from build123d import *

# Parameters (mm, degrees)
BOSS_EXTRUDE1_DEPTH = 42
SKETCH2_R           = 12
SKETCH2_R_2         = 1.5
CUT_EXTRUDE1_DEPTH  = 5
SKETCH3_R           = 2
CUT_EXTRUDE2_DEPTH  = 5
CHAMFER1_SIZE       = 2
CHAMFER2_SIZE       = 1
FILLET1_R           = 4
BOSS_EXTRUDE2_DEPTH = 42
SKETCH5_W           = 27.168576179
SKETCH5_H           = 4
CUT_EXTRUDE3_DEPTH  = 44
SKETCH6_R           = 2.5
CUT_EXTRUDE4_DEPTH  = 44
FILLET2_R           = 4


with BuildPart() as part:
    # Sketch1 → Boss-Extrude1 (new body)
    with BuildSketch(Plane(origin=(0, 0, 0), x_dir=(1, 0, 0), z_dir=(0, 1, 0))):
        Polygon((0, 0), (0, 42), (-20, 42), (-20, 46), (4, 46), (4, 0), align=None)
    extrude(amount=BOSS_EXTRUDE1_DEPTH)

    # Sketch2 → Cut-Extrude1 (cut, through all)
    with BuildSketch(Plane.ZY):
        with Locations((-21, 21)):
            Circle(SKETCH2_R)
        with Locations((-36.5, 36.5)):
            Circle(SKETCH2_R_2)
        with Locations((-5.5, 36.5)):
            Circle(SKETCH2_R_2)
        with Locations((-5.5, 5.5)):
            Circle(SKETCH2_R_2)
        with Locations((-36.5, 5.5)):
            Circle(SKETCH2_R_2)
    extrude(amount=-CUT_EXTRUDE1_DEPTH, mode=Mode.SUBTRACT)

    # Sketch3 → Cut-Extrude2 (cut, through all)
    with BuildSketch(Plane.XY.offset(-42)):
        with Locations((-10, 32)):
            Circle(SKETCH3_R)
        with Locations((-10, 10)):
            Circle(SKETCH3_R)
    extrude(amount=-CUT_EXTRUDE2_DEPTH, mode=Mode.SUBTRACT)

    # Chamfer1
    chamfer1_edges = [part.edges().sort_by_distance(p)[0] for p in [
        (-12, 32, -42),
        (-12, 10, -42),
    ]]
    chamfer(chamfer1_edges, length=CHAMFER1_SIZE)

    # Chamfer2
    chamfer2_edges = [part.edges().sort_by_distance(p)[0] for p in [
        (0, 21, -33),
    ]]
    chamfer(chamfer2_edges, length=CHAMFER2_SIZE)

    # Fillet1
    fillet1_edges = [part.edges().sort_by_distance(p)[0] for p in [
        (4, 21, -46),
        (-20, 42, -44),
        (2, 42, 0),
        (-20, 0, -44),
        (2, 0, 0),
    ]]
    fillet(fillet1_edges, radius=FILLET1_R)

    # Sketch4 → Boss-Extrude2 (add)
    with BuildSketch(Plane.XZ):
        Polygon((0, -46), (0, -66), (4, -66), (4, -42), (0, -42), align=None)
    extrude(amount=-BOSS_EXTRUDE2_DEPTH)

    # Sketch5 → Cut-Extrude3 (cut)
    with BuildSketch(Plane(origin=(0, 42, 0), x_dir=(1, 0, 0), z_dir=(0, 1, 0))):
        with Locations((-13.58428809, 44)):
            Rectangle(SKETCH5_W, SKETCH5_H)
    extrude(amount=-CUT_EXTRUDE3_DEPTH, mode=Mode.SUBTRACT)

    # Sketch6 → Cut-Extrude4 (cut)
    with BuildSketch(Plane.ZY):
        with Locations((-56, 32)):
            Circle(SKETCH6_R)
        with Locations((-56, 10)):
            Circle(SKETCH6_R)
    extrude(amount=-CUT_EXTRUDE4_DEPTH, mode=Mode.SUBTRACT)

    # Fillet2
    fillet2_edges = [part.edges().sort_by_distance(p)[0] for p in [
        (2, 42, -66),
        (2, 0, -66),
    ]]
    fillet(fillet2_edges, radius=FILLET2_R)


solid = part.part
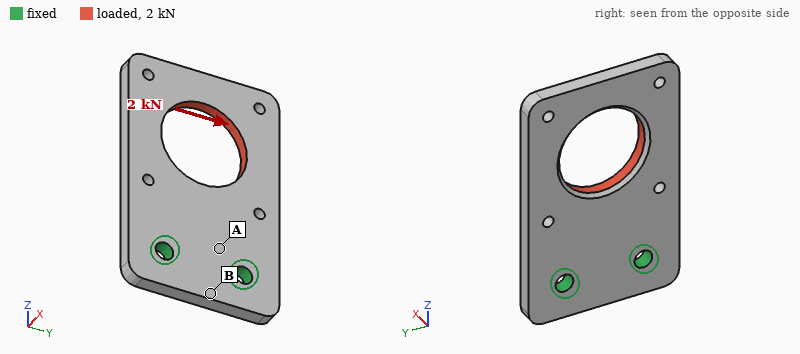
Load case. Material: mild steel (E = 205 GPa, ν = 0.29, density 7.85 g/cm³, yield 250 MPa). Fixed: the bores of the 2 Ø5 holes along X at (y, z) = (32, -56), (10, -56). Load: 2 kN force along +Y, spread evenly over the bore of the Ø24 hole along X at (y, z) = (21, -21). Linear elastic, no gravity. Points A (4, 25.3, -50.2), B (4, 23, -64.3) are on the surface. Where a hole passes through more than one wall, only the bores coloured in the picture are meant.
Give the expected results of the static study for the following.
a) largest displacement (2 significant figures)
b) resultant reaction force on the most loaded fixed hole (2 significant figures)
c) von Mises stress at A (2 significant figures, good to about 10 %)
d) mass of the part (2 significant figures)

40 µm
2.9 kN
44 MPa
70 g
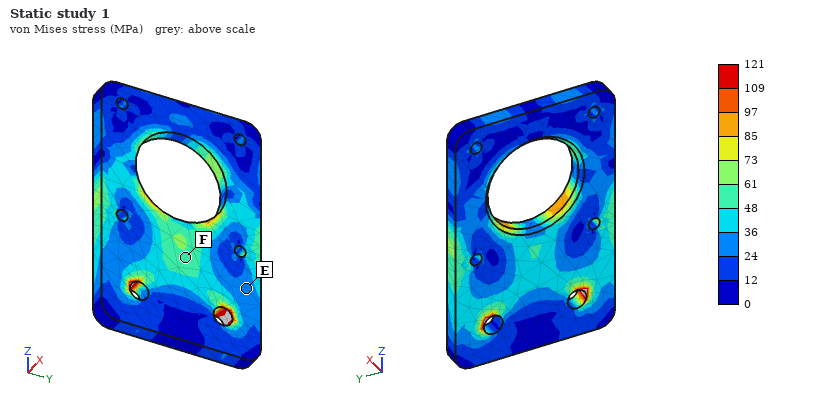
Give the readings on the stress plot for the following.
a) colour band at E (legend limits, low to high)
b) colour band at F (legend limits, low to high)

24 to 36 MPa
48 to 61 MPa
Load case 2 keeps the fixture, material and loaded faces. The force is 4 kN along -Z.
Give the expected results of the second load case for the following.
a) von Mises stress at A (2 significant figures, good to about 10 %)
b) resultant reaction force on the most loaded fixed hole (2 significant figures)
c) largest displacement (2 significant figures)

28 MPa
2.0 kN
71 µm
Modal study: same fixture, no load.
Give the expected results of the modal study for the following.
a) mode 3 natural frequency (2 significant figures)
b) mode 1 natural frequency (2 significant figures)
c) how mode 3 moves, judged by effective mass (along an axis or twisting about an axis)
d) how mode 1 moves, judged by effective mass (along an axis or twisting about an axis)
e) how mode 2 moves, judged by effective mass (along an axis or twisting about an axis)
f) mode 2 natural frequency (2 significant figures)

6000 Hz
1100 Hz
along X
along X
twisting about Z
2800 Hz
